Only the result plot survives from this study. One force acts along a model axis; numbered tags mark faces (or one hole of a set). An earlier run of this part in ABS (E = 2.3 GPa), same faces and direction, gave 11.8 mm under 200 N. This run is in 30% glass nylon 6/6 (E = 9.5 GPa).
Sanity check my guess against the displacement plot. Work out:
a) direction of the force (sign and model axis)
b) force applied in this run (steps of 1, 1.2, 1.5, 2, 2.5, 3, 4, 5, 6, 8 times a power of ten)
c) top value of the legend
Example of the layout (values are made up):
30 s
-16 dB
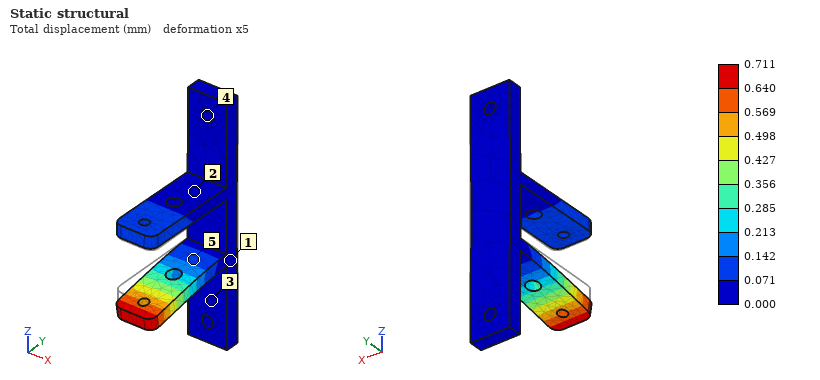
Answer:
-Z
50 N
0.711 mm
